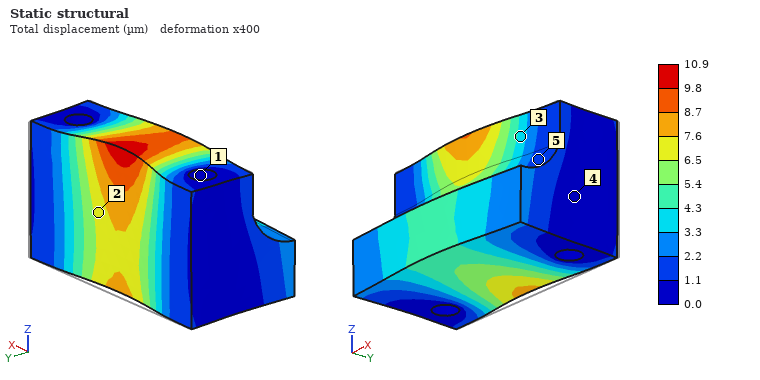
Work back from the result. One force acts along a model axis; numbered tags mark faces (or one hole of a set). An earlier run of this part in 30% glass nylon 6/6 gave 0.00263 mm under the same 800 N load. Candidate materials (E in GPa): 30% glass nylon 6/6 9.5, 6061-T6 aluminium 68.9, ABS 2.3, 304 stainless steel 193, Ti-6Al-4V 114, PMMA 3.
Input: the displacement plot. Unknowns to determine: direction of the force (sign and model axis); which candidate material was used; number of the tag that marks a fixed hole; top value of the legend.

-Y
ABS
1
10.9 µm
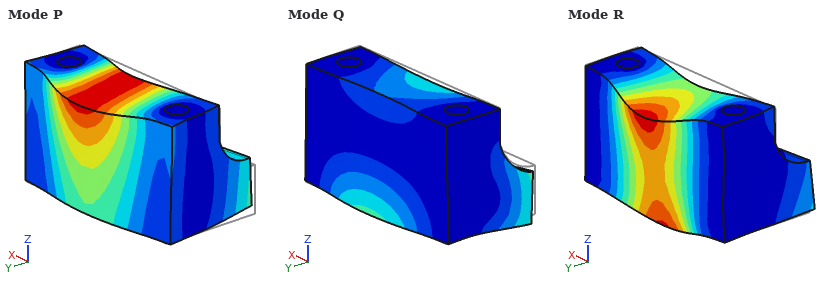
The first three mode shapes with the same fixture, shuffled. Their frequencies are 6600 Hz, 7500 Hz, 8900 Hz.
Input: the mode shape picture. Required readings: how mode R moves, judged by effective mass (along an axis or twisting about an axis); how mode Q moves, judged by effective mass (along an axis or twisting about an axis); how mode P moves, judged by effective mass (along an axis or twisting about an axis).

along Z
along Z
along Y
